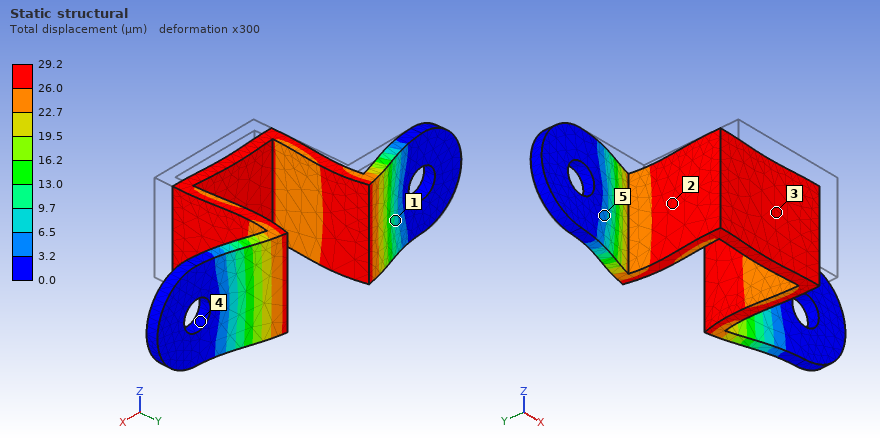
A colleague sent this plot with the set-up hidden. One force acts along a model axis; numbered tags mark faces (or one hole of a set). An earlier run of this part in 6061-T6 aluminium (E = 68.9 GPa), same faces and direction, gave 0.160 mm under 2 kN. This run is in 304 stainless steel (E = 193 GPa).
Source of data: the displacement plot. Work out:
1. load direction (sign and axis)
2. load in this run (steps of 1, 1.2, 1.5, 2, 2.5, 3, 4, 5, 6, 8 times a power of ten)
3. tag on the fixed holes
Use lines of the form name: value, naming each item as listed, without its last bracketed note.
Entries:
load direction: +Y
load in this run: 1 kN
tag on the fixed holes: 4
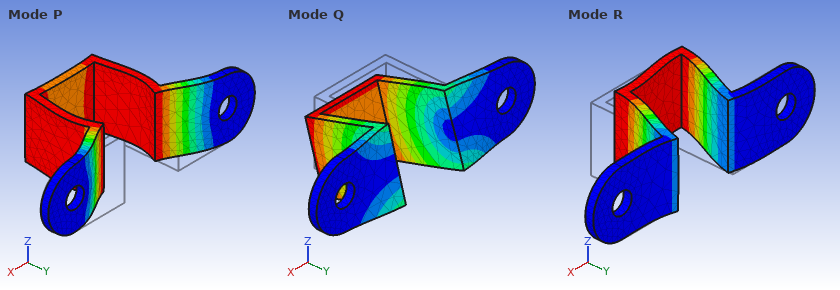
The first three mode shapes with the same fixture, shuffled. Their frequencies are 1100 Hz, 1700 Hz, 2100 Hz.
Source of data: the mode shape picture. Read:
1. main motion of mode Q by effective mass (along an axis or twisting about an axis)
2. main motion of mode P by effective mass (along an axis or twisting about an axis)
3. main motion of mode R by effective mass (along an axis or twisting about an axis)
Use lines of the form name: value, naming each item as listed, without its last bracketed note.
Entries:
main motion of mode Q by effective mass: along Z
main motion of mode P by effective mass: along Y
main motion of mode R by effective mass: along X
